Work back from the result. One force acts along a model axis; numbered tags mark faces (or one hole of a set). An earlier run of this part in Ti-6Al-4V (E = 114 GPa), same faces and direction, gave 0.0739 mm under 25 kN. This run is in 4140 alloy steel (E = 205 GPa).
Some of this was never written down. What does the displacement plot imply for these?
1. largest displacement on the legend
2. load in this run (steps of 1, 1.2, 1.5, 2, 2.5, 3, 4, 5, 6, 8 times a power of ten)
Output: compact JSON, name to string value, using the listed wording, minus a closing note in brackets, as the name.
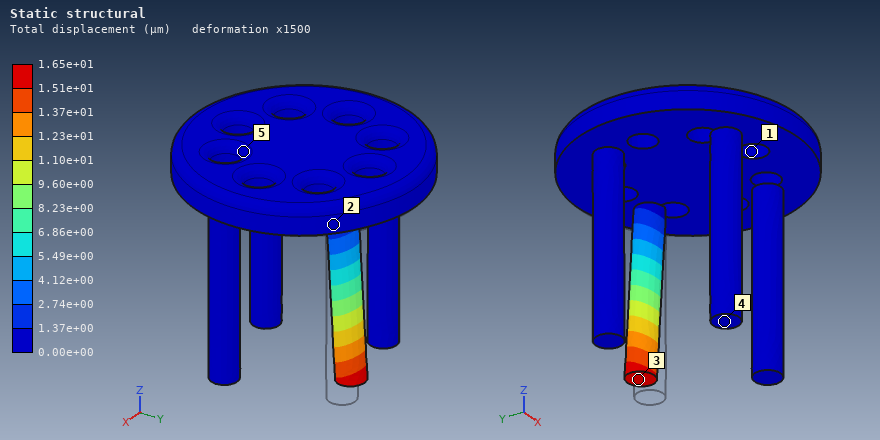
{"largest displacement on the legend": "1.65e+01 µm", "load in this run": "10 kN"}
